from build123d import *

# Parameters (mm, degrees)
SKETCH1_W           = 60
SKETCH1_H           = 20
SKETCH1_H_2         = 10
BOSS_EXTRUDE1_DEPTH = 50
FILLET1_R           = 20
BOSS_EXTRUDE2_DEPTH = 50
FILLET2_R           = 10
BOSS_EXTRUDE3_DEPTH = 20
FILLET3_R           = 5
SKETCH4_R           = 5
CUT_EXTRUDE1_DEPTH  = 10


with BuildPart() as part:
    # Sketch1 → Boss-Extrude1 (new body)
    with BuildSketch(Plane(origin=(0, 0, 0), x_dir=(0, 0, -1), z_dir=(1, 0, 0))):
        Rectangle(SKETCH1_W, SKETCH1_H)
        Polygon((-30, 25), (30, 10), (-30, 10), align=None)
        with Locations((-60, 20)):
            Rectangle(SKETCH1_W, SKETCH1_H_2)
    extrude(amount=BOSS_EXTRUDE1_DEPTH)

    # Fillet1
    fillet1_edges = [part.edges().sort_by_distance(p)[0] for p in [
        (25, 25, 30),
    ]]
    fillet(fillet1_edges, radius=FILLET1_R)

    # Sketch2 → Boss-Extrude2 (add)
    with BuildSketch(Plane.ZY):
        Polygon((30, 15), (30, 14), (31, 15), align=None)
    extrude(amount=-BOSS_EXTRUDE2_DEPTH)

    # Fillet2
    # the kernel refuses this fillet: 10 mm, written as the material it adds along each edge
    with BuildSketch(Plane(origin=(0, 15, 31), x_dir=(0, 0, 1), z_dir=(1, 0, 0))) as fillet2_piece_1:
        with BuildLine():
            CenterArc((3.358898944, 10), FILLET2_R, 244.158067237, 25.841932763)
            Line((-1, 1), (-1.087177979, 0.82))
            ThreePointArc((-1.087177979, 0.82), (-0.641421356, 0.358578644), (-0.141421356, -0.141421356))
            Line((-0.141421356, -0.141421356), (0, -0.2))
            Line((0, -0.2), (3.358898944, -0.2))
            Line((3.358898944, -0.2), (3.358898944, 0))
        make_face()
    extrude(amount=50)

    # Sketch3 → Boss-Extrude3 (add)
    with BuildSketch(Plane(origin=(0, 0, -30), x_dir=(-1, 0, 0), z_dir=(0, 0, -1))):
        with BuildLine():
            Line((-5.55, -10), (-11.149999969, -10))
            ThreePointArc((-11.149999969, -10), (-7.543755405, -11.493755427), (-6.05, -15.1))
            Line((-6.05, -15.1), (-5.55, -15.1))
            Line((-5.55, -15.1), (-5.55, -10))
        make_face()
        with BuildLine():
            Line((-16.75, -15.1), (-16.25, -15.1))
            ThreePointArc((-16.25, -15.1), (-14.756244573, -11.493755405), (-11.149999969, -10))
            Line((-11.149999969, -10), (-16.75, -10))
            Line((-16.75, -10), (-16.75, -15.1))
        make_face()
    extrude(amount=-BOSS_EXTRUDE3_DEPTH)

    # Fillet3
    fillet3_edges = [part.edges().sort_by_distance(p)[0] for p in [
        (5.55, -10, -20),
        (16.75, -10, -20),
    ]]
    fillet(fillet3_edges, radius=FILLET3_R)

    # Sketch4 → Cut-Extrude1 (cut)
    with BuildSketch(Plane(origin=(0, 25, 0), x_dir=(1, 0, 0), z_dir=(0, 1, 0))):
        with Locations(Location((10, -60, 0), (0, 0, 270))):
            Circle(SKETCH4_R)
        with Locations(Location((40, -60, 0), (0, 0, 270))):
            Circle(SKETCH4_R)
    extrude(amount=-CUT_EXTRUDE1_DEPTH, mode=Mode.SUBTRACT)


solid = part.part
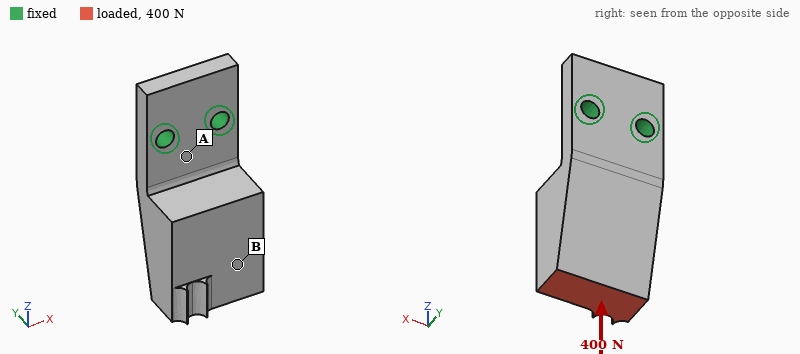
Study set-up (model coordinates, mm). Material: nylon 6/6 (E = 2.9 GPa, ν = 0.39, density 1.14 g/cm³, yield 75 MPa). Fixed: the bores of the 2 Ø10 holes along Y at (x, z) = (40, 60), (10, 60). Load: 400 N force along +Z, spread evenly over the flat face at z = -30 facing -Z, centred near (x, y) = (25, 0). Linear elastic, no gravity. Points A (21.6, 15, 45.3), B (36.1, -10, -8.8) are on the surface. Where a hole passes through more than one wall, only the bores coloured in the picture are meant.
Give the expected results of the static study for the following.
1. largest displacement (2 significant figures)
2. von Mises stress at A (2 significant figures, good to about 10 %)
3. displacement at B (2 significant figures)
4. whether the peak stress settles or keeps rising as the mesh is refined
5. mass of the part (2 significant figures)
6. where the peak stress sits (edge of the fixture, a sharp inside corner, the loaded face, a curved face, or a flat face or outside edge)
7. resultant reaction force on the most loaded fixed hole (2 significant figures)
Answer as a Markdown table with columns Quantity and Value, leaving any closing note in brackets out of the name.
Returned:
| Quantity | Value |
|---|---|
| largest displacement | 1.6 mm |
| von Mises stress at A | 9.0 MPa |
| displacement at B | 1.2 mm |
| whether the peak stress settles or keeps rising as the mesh is refined | keeps rising |
| mass of the part | 130 g |
| where the peak stress sits | edge of the fixture |
| resultant reaction force on the most loaded fixed hole | 210 N |
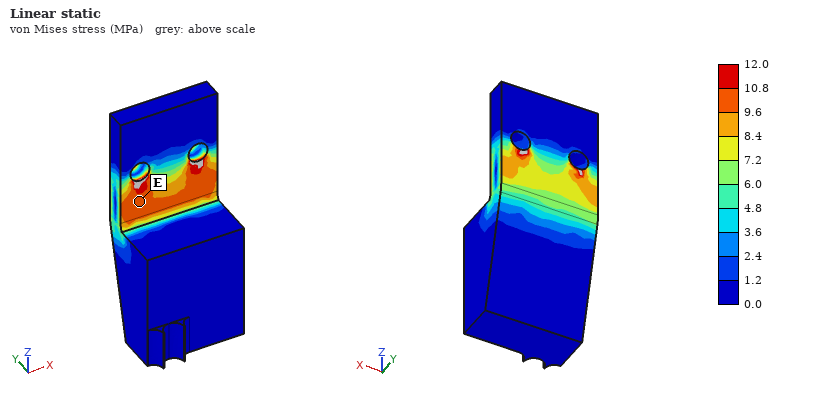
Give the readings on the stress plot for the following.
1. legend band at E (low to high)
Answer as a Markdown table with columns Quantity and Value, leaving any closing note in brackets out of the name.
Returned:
| Quantity | Value |
|---|---|
| legend band at E | 9.6 to 10.8 MPa |
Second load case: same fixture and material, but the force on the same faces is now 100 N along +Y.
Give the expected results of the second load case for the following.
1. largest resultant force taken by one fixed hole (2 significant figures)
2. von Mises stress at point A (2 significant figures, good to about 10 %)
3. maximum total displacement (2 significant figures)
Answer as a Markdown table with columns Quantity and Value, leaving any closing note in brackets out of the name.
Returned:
| Quantity | Value |
|---|---|
| largest resultant force taken by one fixed hole | 52 N |
| von Mises stress at point A | 7.7 MPa |
| maximum total displacement | 1.5 mm |
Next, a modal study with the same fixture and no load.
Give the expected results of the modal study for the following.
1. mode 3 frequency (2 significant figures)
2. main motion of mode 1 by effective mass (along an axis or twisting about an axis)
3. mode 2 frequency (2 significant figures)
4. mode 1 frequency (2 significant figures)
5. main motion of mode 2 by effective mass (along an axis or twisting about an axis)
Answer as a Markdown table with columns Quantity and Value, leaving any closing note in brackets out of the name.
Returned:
| Quantity | Value |
|---|---|
| mode 3 frequency | 1200 Hz |
| main motion of mode 1 by effective mass | along Y |
| mode 2 frequency | 660 Hz |
| mode 1 frequency | 220 Hz |
| main motion of mode 2 by effective mass | along X |
